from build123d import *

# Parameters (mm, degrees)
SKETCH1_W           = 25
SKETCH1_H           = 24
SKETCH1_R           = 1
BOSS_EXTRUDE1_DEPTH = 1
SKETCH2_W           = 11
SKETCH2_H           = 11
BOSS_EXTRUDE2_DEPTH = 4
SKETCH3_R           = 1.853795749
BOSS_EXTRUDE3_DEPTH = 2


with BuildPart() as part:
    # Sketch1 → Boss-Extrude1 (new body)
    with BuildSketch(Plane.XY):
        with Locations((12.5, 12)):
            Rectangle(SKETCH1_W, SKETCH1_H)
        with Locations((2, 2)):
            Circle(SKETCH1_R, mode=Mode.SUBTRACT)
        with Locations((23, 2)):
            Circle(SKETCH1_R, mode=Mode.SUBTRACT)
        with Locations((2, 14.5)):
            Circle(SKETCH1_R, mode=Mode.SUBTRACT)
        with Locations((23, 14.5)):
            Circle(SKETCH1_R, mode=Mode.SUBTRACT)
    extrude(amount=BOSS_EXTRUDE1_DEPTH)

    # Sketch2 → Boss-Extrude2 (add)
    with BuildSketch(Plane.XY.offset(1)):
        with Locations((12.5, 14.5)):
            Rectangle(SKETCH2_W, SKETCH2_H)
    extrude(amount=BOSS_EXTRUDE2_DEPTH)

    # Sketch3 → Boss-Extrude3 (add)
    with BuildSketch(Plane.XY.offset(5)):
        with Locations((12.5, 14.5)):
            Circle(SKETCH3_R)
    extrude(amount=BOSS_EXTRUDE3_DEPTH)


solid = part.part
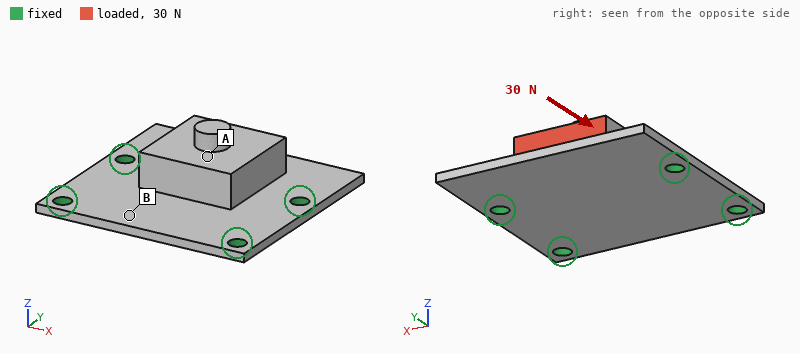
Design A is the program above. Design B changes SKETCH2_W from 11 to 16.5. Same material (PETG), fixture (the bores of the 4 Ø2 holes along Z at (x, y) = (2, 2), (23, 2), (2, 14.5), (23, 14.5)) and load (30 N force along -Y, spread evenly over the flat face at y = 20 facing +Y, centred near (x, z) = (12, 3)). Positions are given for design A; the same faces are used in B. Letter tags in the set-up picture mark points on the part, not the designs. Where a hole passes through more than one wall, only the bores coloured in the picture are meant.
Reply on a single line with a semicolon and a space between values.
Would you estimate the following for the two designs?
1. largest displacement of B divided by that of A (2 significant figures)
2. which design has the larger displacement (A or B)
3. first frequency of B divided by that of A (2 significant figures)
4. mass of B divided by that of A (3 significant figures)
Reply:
0.51; A; 1.3; 1.22
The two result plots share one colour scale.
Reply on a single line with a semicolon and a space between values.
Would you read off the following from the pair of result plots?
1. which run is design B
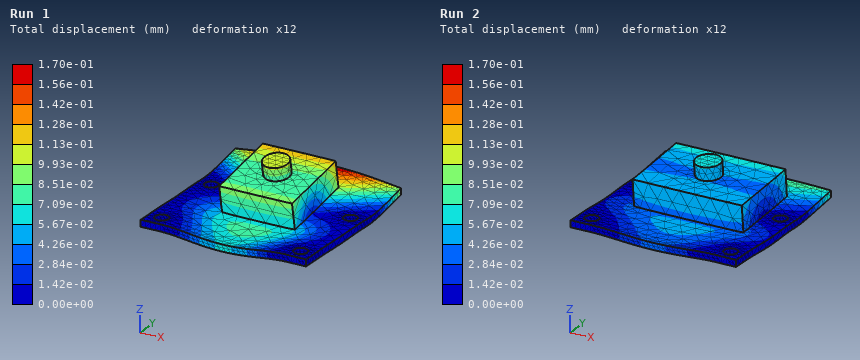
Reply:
Run 2
